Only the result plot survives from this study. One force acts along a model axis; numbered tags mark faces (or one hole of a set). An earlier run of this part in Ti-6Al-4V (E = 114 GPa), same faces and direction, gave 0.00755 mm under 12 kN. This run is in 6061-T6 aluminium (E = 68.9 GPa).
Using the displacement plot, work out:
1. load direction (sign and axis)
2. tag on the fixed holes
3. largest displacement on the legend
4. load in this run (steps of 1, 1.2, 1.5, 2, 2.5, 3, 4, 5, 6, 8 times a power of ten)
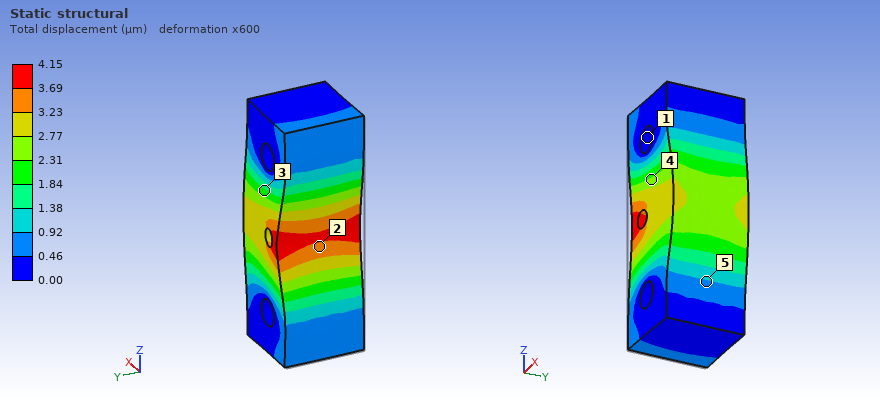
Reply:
+X
1
4.15 µm
4 kN
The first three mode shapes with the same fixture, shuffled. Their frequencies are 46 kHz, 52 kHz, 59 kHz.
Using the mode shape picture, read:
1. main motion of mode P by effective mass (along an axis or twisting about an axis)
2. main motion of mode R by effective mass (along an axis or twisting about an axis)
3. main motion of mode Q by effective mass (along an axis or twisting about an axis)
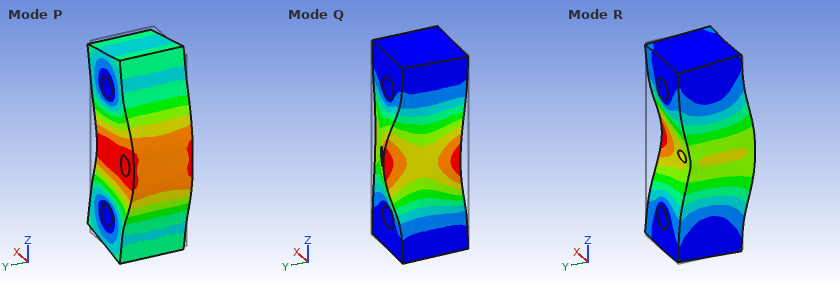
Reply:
along X
along Y
twisting about Z
